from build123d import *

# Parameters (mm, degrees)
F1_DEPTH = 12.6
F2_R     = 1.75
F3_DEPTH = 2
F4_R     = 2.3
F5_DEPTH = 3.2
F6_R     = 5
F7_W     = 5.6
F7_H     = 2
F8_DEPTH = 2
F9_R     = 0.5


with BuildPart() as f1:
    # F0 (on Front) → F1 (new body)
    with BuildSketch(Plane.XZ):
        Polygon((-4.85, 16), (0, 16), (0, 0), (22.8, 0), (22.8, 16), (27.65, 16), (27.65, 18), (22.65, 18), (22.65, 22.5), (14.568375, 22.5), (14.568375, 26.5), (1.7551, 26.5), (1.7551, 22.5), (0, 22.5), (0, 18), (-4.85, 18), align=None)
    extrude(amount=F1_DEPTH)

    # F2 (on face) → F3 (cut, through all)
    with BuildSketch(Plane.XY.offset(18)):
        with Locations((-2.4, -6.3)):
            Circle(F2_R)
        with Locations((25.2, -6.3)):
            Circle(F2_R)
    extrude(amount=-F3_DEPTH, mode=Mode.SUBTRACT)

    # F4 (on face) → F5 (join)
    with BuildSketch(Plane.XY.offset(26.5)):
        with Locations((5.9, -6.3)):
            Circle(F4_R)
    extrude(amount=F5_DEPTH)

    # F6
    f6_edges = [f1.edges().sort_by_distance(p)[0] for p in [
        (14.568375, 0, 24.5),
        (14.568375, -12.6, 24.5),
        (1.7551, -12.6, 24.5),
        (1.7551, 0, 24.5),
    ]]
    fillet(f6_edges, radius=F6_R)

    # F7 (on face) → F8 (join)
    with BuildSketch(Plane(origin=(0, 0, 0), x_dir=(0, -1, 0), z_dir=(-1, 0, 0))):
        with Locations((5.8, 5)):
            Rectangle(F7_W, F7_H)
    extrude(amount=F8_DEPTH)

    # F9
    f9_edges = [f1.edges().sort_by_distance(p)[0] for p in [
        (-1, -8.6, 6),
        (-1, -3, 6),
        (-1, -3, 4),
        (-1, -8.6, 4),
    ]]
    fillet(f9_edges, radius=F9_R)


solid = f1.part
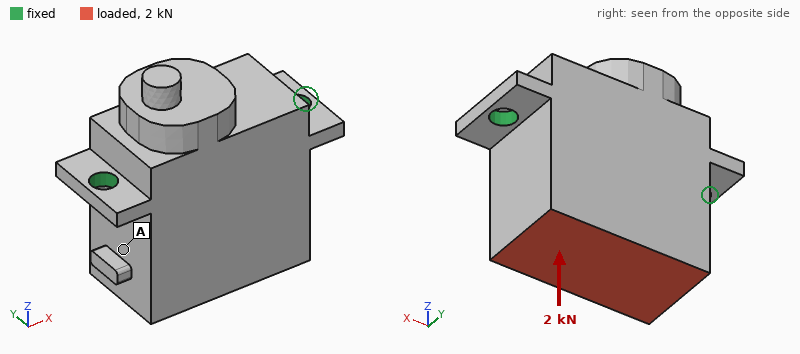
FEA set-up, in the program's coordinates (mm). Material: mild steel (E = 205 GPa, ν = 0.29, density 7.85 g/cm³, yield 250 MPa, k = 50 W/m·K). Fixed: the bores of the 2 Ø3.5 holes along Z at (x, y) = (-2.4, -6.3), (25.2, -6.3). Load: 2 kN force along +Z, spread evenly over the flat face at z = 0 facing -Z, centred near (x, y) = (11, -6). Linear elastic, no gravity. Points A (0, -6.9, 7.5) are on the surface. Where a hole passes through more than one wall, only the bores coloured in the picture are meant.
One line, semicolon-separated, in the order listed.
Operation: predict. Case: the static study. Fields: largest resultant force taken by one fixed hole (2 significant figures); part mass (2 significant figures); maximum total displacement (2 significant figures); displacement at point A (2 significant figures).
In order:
1.0 kN; 57 g; 3.3 µm; 2.9 µm
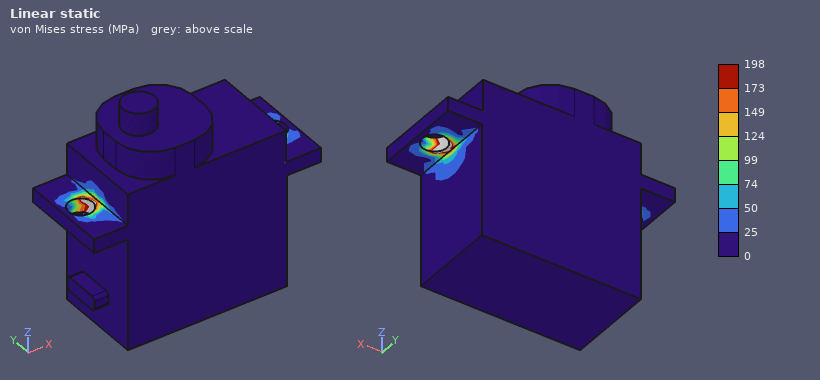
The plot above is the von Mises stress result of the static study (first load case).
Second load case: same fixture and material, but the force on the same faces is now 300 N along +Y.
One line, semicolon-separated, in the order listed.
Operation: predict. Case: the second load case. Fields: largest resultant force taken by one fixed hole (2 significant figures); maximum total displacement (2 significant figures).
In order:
150 N; 26 µm
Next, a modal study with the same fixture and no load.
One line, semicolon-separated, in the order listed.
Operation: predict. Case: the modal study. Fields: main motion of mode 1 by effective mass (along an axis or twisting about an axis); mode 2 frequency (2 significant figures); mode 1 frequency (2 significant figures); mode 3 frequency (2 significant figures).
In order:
along Y; 18 kHz; 4400 Hz; 18 kHz
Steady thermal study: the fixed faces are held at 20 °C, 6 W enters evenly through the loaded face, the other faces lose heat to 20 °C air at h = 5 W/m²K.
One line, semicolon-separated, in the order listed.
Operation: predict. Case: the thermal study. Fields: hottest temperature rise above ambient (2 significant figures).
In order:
15 K
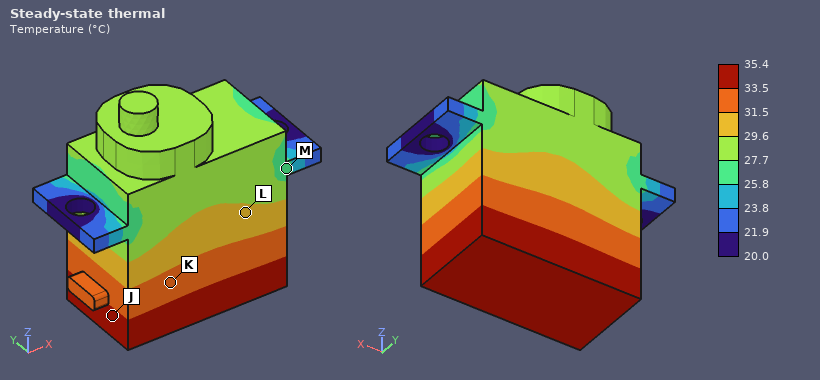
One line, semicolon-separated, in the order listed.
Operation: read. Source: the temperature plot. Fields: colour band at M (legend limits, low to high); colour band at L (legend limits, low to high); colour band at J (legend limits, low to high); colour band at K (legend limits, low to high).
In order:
25.8 to 27.7 °C; 29.6 to 31.5 °C; 33.5 to 35.4 °C; 31.5 to 33.5 °C
